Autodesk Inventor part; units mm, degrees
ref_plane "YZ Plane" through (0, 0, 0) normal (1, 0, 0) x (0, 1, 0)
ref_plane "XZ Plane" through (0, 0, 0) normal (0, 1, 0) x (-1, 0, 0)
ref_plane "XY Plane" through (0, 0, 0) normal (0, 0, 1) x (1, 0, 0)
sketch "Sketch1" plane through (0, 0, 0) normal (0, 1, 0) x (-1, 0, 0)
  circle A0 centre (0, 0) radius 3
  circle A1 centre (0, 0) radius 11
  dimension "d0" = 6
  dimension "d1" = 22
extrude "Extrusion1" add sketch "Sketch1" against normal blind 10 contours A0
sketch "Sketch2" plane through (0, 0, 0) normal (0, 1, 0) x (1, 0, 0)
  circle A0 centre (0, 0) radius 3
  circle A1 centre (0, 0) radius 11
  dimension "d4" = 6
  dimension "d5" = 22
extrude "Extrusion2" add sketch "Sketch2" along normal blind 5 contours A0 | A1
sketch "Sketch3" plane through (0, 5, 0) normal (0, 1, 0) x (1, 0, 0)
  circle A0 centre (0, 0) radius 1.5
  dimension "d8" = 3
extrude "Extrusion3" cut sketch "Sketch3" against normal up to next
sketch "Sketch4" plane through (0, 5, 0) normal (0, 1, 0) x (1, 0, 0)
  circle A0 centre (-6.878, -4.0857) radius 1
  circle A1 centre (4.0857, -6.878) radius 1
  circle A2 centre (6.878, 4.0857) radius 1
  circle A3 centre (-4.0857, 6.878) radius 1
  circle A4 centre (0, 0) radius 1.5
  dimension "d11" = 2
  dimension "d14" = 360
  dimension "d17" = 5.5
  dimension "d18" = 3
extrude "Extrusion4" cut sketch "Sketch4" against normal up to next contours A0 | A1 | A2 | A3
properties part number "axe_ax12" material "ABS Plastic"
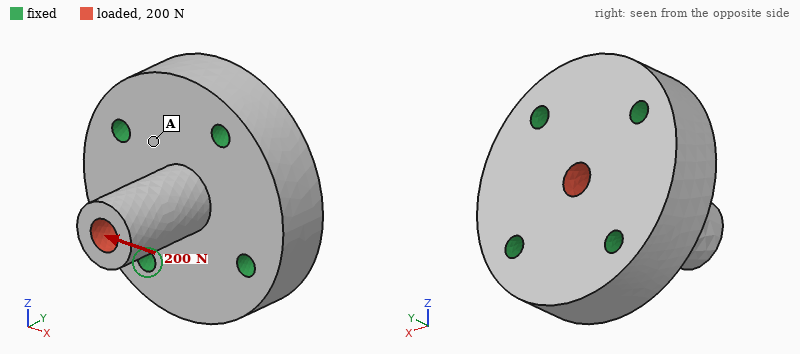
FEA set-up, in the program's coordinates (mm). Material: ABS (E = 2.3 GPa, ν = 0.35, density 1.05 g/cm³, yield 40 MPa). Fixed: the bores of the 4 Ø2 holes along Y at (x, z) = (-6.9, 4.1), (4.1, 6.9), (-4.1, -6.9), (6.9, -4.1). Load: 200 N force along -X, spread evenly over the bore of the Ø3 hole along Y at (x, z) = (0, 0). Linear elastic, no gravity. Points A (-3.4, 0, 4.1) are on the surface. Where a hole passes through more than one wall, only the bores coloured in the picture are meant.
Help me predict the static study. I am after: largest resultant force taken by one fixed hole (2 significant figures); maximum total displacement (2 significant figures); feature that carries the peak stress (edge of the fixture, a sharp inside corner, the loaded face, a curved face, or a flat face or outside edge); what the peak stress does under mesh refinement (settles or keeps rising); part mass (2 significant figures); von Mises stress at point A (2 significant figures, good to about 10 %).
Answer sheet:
84 N
0.28 mm
a sharp inside corner
keeps rising
2.1 g
3.7 MPa
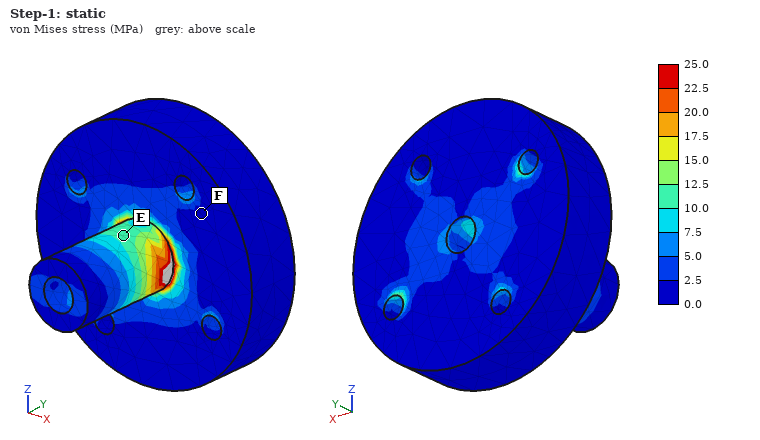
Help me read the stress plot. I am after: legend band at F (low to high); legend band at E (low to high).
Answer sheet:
0.0 to 2.5 MPa
10.0 to 12.5 MPa
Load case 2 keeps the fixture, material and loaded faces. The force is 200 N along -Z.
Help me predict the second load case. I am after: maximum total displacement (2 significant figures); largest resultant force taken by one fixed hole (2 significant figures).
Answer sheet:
0.28 mm
84 N
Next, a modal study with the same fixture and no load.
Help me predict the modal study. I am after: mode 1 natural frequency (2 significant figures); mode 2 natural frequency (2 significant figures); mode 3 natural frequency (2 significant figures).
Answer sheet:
8800 Hz
8800 Hz
21 kHz
